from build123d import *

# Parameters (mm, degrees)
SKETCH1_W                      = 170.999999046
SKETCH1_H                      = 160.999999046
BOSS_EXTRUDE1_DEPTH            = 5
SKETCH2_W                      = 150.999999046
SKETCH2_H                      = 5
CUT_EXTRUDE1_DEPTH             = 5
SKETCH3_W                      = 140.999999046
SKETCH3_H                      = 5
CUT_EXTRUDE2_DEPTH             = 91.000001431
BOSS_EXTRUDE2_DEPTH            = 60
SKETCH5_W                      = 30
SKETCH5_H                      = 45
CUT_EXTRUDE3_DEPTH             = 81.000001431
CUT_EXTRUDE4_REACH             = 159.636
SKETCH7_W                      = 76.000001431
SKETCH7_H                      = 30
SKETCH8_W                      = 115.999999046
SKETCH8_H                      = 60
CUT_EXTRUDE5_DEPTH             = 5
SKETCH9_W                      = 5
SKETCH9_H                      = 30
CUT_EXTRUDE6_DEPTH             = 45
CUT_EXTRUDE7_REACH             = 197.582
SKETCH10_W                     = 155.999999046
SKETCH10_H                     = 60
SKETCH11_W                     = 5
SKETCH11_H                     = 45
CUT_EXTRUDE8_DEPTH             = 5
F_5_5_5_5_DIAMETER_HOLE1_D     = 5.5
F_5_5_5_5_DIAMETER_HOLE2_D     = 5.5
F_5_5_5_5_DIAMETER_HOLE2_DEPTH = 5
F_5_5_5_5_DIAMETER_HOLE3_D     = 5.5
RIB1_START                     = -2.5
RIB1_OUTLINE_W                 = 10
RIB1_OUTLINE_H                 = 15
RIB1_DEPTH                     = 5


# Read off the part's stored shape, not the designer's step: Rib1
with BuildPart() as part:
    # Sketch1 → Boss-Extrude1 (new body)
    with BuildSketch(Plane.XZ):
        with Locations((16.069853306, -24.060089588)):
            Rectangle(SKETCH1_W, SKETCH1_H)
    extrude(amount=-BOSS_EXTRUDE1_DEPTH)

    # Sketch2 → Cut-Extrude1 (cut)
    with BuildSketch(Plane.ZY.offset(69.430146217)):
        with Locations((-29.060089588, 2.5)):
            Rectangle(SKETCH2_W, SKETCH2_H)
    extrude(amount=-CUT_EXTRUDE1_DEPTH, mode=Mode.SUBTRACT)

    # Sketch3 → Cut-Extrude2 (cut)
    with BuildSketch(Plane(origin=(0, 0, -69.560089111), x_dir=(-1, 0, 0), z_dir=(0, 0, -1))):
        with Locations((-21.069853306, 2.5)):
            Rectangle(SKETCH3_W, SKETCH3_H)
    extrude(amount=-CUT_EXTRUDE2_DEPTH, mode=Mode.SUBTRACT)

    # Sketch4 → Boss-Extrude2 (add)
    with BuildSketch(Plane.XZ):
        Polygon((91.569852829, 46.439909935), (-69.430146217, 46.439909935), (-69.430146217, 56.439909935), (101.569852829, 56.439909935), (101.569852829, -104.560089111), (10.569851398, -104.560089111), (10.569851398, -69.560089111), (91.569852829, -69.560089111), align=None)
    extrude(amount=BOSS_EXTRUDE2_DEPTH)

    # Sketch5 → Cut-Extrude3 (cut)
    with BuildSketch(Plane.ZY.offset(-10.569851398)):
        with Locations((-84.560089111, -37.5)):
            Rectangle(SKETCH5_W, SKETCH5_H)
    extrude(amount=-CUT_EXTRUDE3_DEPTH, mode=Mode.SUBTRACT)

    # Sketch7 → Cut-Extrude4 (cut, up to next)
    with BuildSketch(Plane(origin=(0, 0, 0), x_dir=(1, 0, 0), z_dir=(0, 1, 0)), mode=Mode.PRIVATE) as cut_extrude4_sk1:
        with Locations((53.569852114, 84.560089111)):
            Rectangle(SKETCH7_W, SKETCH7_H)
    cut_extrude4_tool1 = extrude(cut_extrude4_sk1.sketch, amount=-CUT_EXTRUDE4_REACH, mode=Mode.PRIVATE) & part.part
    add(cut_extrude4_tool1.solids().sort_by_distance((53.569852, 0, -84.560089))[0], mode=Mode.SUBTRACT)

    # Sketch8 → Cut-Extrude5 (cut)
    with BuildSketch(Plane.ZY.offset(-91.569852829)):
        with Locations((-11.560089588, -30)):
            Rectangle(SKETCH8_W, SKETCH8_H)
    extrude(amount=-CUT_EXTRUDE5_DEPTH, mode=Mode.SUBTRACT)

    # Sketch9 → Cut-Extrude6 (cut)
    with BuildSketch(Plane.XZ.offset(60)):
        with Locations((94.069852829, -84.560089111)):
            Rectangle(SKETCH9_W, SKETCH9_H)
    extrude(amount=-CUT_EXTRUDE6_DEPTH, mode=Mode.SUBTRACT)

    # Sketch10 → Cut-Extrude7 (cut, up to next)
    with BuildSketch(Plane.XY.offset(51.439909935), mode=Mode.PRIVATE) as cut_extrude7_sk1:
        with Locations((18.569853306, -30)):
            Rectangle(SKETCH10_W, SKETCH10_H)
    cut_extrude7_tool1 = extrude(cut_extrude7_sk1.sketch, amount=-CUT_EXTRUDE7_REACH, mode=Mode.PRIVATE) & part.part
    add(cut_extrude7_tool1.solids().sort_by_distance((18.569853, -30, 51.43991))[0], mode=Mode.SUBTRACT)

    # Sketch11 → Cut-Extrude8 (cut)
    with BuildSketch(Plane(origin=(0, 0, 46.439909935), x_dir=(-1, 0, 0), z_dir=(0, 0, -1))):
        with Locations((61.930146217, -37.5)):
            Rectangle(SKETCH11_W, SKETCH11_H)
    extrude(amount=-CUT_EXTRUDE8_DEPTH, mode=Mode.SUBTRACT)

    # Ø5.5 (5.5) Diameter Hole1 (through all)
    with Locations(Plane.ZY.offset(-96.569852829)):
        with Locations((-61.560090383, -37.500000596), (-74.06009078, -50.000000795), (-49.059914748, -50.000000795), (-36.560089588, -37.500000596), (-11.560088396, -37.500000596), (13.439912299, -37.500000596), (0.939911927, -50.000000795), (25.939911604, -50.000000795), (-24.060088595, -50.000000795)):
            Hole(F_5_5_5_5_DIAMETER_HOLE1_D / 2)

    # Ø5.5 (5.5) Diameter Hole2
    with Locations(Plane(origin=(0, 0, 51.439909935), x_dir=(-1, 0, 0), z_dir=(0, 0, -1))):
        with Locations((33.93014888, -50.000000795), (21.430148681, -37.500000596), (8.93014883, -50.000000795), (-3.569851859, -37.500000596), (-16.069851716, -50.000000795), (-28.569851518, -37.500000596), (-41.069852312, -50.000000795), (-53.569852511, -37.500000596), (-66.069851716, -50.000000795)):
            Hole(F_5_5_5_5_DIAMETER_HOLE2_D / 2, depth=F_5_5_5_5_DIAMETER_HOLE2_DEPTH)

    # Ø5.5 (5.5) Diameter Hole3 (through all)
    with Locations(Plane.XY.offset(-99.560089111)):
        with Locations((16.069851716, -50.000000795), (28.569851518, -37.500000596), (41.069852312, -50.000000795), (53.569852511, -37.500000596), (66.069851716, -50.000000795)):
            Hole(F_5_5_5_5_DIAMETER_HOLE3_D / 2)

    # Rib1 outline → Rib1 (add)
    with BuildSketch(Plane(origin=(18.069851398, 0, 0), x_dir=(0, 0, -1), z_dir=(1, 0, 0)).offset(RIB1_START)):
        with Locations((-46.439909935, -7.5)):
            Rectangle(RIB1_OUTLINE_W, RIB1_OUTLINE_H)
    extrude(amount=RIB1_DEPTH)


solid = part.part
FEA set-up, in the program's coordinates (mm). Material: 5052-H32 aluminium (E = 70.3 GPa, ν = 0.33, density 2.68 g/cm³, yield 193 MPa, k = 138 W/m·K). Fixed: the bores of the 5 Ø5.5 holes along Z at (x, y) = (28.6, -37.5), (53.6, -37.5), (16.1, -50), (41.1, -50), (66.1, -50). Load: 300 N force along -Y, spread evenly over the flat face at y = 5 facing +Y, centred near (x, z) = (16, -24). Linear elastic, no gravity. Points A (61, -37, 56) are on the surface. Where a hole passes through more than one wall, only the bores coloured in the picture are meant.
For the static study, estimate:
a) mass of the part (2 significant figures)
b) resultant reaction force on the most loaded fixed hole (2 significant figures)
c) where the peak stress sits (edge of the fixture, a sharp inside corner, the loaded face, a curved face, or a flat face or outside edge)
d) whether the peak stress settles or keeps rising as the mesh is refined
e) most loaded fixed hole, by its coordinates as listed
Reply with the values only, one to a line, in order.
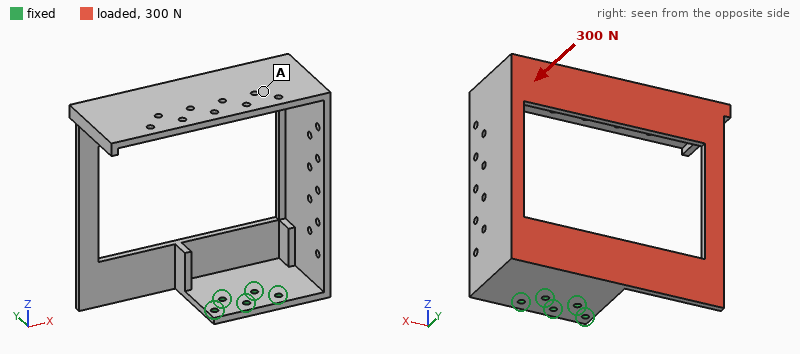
530 g
810 N
edge of the fixture
keeps rising
(53.6, -37.5)
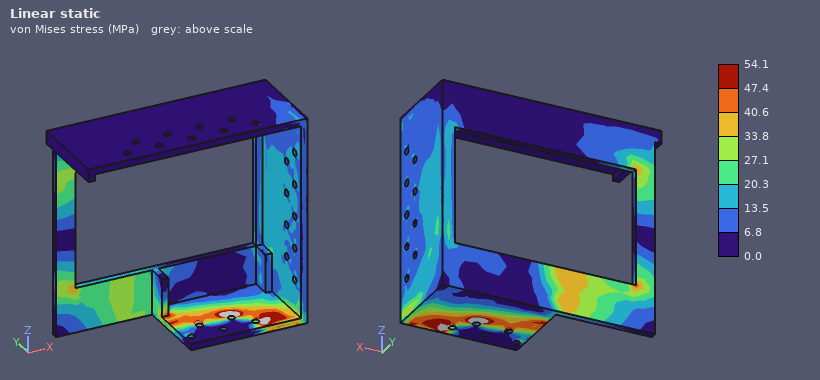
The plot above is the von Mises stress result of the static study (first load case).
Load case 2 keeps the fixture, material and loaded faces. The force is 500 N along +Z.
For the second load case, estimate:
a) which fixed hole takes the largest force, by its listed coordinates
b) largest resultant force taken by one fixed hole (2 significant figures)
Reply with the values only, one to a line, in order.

(28.6, -37.5)
710 N
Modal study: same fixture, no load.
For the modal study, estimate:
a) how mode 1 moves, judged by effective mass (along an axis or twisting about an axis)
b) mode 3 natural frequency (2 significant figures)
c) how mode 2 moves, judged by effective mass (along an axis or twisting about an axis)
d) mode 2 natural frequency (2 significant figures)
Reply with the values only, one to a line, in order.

along Y
290 Hz
along X
120 Hz
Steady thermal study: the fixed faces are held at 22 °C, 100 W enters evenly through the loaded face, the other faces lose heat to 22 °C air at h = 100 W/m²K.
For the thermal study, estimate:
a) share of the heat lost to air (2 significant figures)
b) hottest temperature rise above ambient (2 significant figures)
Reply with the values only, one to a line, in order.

83 %
33 K
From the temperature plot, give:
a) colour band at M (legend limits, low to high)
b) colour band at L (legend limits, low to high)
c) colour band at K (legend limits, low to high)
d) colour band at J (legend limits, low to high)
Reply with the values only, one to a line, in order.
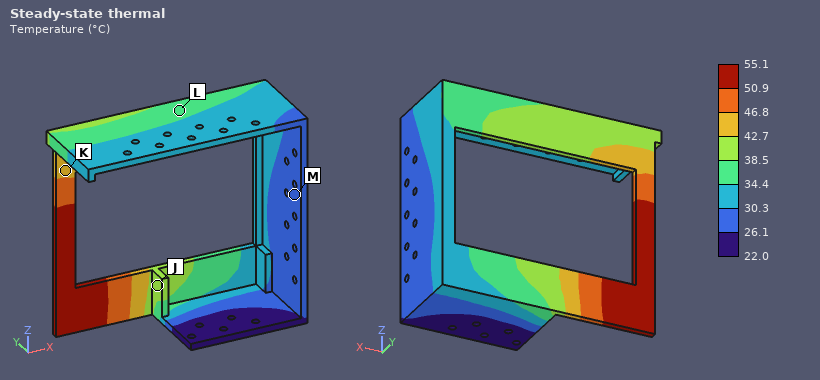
26.1 to 30.3 °C
34.4 to 38.5 °C
42.7 to 46.8 °C
38.5 to 42.7 °C
